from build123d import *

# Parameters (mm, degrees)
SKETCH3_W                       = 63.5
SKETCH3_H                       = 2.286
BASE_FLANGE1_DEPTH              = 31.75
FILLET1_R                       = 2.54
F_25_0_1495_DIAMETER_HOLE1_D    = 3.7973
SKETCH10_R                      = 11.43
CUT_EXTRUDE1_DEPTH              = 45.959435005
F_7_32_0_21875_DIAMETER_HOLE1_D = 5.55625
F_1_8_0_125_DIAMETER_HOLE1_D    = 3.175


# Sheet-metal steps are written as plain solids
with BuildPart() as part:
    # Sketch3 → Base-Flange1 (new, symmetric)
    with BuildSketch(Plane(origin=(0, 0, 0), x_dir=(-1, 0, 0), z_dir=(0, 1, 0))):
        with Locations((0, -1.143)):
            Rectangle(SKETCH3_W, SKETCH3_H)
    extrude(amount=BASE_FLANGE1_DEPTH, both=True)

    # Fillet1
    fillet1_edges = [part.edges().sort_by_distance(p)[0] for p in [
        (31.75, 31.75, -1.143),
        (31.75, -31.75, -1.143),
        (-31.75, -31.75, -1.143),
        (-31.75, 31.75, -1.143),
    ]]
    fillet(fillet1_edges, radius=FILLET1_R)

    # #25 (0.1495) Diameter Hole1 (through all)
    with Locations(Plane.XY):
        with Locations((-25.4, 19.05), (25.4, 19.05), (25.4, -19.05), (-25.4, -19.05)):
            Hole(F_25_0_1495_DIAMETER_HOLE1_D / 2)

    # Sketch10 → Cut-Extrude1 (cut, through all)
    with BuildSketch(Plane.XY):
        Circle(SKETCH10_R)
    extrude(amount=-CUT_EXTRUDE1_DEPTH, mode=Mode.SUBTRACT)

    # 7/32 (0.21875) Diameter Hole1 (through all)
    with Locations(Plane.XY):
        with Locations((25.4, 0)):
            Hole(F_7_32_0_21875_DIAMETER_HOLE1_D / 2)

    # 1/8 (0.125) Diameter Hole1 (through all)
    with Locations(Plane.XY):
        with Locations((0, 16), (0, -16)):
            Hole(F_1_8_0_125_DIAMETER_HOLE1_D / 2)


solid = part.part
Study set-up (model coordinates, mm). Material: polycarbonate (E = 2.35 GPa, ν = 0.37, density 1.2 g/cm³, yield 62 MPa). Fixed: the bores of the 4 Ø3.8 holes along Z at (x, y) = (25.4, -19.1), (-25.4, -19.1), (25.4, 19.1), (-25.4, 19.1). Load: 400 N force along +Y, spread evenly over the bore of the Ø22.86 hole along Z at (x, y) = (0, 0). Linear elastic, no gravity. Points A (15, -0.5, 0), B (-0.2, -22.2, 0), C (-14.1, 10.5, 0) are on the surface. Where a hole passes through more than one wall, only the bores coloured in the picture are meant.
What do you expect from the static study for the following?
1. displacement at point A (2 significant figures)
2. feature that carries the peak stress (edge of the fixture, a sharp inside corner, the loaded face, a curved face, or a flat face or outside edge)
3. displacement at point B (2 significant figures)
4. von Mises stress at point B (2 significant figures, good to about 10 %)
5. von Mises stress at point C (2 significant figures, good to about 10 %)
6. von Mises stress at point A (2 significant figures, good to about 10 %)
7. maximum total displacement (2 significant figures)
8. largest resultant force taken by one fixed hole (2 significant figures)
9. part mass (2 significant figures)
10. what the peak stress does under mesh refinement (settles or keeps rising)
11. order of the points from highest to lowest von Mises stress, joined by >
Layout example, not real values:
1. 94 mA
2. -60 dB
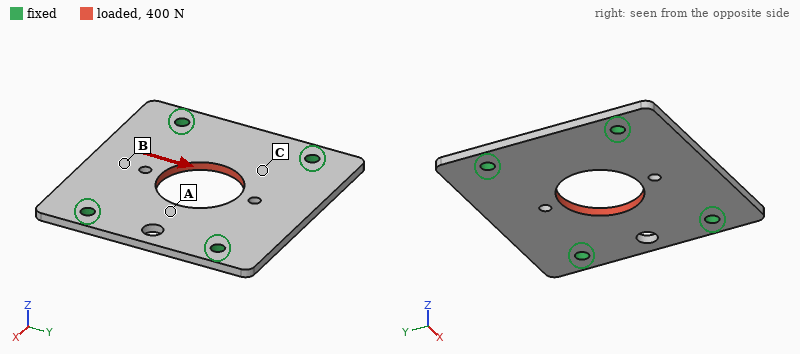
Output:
1. 30 µm
2. edge of the fixture
3. 46 µm
4. 1.2 MPa
5. 2.7 MPa
6. 4.5 MPa
7. 57 µm
8. 110 N
9. 9.7 g
10. keeps rising
11. A > C > B
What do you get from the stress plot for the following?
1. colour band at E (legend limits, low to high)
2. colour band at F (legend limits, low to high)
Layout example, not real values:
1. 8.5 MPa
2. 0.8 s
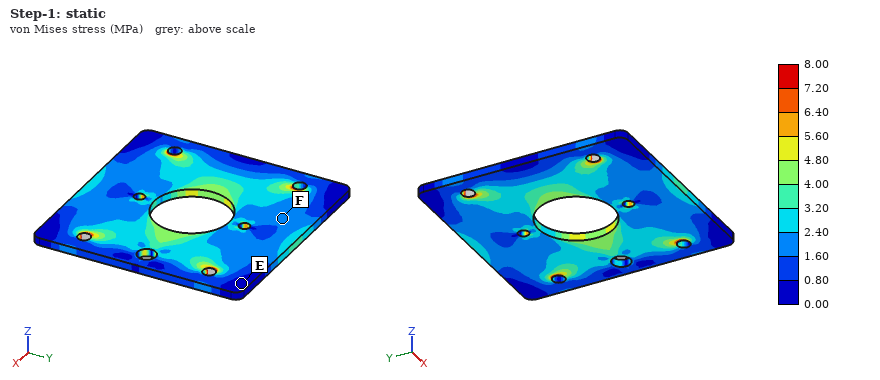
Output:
1. 0.00 to 0.80 MPa
2. 1.60 to 2.40 MPa
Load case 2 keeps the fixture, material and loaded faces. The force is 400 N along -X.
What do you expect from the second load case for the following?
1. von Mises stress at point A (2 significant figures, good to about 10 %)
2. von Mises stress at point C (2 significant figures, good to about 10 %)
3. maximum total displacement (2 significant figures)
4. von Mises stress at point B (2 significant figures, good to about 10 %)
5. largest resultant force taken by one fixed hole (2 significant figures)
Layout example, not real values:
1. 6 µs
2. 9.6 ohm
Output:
1. 1.9 MPa
2. 2.6 MPa
3. 38 µm
4. 1.2 MPa
5. 110 N
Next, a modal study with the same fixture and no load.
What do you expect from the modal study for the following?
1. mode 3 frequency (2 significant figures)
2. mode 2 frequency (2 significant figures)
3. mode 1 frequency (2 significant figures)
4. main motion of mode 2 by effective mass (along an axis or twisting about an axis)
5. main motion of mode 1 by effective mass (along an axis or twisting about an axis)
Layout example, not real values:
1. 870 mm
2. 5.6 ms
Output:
1. 1600 Hz
2. 1300 Hz
3. 1200 Hz
4. twisting about X
5. along Z
